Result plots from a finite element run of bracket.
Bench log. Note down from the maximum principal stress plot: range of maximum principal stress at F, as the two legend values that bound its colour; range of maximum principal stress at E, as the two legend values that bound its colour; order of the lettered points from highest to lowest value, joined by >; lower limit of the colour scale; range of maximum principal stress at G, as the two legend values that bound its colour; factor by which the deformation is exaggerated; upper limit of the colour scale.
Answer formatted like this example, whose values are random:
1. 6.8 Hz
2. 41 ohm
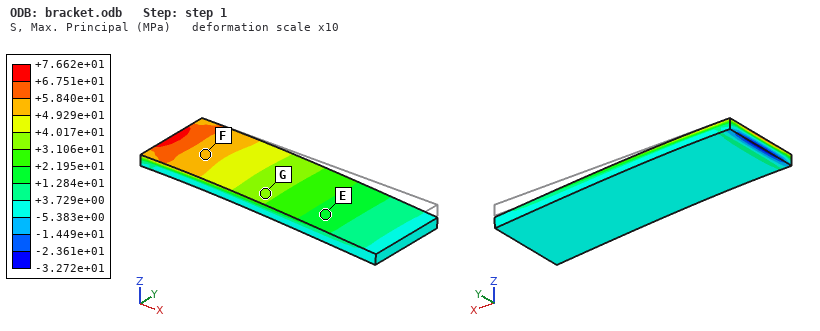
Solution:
1. +4.929e+01 to +5.840e+01 MPa
2. +1.284e+01 to +2.195e+01 MPa
3. F > G > E
4. -3.272e+01 MPa
5. +3.106e+01 to +4.017e+01 MPa
6. 10
7. +7.662e+01 MPa
